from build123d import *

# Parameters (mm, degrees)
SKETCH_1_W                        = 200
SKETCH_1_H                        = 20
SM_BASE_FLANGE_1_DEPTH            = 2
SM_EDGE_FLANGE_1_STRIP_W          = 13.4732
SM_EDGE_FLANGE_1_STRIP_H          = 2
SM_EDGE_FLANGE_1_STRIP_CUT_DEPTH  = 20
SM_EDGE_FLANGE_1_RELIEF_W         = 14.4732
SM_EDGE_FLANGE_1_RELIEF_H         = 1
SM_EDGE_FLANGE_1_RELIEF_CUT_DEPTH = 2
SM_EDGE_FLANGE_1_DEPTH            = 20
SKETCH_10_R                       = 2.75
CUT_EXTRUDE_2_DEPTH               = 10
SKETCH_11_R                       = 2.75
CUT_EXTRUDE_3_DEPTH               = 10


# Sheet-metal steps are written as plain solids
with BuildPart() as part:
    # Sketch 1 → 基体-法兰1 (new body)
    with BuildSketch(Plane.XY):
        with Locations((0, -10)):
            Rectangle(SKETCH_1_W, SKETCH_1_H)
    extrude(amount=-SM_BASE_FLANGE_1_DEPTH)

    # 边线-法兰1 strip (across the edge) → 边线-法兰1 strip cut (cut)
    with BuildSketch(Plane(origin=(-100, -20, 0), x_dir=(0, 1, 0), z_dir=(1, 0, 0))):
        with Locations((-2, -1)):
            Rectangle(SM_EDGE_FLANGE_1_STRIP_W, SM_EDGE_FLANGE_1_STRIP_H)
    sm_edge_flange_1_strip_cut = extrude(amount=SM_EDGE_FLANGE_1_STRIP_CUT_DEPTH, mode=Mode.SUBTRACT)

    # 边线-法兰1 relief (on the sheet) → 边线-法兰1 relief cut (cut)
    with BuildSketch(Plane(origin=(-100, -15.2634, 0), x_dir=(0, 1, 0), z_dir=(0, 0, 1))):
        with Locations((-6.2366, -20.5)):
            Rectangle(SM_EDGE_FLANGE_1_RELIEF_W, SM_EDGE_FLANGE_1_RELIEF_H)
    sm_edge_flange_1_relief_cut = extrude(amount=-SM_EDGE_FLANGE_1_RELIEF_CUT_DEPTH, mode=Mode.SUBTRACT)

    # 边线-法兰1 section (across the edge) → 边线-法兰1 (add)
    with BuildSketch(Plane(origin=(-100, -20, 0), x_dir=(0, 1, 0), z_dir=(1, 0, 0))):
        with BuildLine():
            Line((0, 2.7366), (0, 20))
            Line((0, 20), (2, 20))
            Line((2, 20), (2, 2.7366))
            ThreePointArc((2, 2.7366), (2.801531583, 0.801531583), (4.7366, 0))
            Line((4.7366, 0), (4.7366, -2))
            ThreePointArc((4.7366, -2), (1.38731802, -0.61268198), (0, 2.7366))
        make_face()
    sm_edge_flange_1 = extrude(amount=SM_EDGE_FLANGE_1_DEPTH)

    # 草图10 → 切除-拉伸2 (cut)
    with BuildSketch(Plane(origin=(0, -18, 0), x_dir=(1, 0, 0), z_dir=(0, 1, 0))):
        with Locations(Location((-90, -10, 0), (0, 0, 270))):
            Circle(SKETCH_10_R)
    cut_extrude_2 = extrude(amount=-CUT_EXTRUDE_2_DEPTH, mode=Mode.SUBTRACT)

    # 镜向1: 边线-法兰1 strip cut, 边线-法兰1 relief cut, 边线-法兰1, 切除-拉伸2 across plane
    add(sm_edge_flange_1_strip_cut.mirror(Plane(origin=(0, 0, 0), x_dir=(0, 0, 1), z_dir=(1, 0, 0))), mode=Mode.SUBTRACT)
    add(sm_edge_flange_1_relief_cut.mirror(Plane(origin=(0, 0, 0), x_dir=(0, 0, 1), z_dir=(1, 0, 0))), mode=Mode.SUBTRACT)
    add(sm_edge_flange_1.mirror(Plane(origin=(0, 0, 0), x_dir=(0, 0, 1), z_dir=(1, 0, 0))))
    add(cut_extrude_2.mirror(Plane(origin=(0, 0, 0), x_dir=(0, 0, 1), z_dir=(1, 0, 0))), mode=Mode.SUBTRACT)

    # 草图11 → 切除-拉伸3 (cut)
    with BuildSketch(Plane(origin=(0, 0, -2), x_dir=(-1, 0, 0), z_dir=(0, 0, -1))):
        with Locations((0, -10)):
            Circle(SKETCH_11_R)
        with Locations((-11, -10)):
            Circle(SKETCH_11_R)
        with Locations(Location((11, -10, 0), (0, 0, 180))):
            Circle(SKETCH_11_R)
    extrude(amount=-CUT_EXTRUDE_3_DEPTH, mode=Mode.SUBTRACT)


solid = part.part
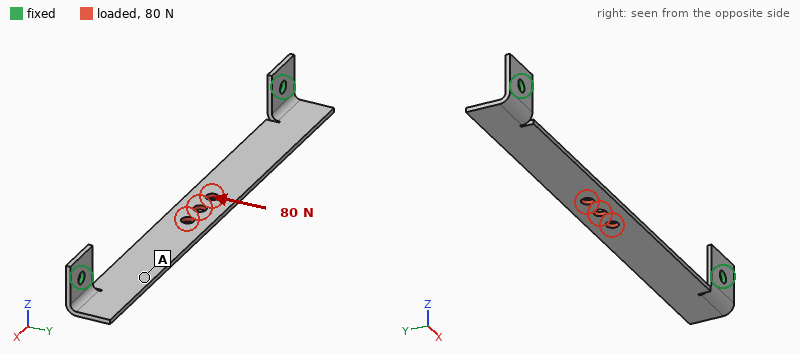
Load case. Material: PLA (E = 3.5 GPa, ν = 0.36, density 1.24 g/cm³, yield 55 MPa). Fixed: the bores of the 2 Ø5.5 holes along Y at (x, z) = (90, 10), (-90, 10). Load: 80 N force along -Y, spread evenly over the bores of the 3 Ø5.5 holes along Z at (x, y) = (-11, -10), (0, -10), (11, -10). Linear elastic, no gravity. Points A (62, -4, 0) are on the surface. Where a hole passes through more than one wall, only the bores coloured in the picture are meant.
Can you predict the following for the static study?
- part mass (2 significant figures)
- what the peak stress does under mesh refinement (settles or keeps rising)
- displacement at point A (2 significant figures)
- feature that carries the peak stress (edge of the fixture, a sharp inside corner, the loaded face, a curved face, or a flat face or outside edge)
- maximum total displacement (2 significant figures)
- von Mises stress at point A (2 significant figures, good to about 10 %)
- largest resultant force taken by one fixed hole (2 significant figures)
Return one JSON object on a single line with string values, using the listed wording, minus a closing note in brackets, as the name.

{"part mass": "11 g", "what the peak stress does under mesh refinement": "keeps rising", "displacement at point A": "1.2 mm", "feature that carries the peak stress": "edge of the fixture", "maximum total displacement": "2.1 mm", "von Mises stress at point A": "4.1 MPa", "largest resultant force taken by one fixed hole": "92 N"}
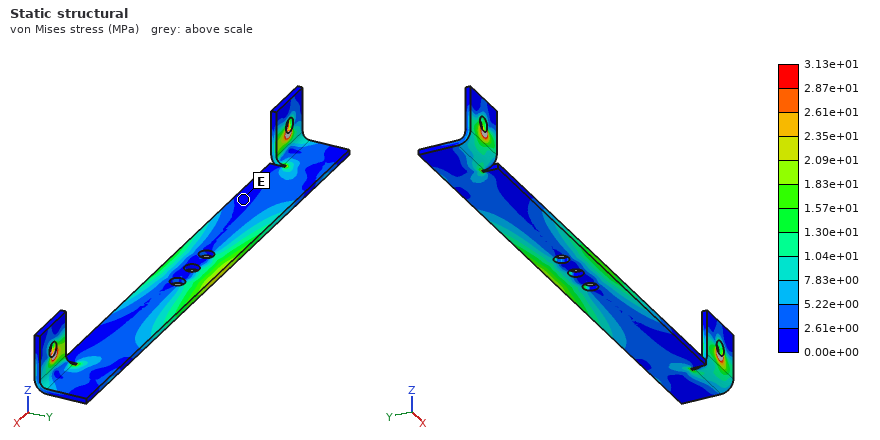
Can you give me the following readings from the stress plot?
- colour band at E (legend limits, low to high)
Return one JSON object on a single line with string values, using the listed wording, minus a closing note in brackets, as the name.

{"colour band at E": "0.00e+00 to 2.61e+00 MPa"}
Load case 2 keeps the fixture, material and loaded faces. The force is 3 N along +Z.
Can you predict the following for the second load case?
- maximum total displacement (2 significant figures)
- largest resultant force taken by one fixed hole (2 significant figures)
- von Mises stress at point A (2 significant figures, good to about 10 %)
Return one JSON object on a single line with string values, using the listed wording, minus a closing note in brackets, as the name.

{"maximum total displacement": "2.2 mm", "largest resultant force taken by one fixed hole": "1.5 N", "von Mises stress at point A": "1.8 MPa"}
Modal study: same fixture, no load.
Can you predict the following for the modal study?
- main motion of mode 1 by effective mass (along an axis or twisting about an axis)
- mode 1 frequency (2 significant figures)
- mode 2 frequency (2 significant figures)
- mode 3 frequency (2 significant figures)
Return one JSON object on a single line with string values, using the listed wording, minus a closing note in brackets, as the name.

{"main motion of mode 1 by effective mass": "along Z", "mode 1 frequency": "100 Hz", "mode 2 frequency": "290 Hz", "mode 3 frequency": "390 Hz"}
